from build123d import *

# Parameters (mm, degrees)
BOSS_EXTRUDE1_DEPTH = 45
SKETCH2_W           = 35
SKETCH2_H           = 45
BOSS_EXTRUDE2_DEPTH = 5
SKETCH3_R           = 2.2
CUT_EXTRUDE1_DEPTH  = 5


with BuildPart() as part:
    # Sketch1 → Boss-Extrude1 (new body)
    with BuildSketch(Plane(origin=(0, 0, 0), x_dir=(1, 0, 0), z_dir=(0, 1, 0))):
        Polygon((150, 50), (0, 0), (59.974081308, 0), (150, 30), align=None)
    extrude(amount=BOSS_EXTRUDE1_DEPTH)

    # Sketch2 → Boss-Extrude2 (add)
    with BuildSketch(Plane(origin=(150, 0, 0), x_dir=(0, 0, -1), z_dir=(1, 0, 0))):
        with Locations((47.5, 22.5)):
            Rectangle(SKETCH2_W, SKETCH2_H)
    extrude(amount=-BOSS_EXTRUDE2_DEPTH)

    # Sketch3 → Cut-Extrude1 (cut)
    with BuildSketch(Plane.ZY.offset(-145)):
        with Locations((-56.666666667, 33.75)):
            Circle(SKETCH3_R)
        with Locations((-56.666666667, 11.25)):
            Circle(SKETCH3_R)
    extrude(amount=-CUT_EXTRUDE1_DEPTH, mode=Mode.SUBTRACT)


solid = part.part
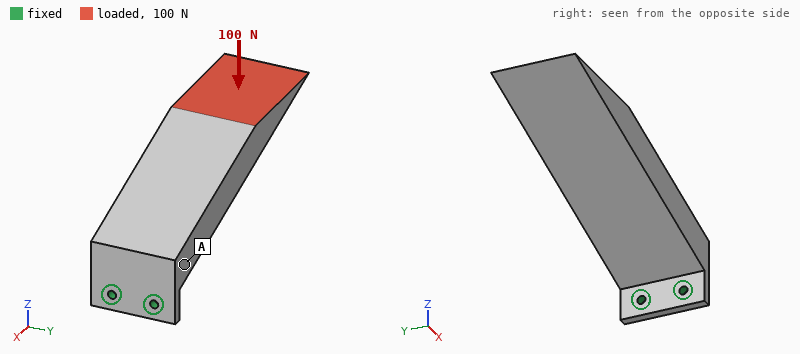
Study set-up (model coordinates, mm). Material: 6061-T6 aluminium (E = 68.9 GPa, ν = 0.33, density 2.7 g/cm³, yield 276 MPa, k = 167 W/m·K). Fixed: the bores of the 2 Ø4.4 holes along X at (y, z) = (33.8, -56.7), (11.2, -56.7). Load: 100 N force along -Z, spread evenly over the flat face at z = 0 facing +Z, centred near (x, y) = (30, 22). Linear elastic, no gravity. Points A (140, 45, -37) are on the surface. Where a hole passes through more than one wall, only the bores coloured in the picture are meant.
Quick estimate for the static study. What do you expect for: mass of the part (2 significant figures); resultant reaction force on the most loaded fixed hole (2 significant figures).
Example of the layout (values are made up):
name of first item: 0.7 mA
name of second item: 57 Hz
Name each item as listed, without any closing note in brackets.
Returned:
mass of the part: 300 g
resultant reaction force on the most loaded fixed hole: 56 N
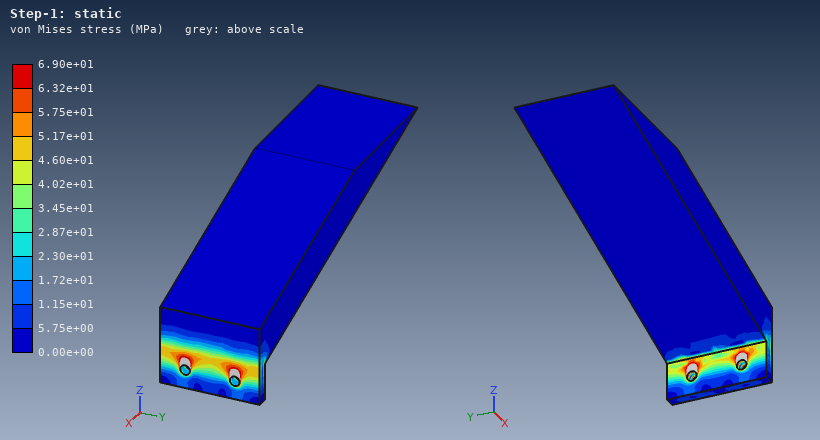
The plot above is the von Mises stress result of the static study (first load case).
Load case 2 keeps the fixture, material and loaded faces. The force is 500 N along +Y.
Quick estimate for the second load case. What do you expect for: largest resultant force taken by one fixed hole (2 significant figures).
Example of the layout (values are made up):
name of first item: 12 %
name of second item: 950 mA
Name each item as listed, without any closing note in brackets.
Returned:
largest resultant force taken by one fixed hole: 2.4 kN
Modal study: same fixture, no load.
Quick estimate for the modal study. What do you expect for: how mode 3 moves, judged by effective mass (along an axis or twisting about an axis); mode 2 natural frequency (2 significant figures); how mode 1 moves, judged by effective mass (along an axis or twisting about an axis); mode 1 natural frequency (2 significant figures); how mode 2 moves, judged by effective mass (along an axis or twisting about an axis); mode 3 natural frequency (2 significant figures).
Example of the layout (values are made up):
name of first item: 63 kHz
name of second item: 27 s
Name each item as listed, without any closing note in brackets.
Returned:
how mode 3 moves, judged by effective mass: along X
mode 2 natural frequency: 600 Hz
how mode 1 moves, judged by effective mass: along Z
mode 1 natural frequency: 200 Hz
how mode 2 moves, judged by effective mass: along Y
mode 3 natural frequency: 2800 Hz
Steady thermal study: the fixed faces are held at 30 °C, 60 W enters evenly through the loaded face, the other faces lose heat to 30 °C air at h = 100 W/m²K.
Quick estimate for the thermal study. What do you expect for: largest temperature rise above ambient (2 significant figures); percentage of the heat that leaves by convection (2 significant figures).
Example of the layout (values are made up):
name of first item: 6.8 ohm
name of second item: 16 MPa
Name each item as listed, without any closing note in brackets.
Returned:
largest temperature rise above ambient: 49 K
percentage of the heat that leaves by convection: 63 %
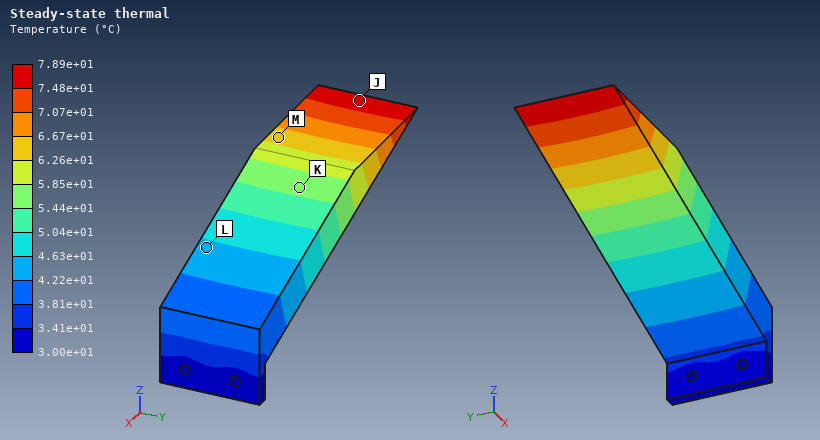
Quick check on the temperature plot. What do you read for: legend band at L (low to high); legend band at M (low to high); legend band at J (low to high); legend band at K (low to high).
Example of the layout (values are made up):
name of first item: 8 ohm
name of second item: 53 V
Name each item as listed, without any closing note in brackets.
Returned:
legend band at L: 4.22e+01 to 4.63e+01 °C
legend band at M: 6.26e+01 to 6.67e+01 °C
legend band at J: 7.48e+01 to 7.89e+01 °C
legend band at K: 5.44e+01 to 5.85e+01 °C
